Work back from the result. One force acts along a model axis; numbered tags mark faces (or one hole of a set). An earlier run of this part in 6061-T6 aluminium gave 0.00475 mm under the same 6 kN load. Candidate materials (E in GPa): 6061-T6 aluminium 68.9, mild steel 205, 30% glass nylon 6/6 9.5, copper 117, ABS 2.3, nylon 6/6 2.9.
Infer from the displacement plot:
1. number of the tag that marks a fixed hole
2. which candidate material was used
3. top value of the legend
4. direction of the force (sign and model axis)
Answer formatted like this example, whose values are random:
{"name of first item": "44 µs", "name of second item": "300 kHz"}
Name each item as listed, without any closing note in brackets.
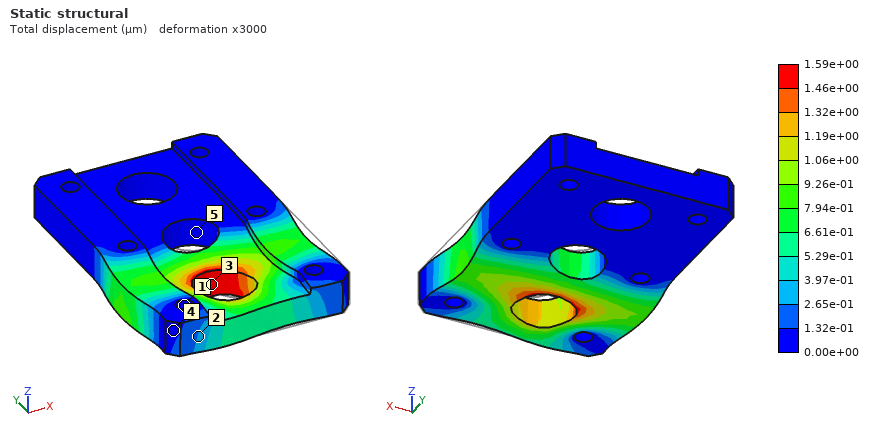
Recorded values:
{"number of the tag that marks a fixed hole": "1", "which candidate material was used": "mild steel", "top value of the legend": "1.59e+00 µm", "direction of the force": "-X"}
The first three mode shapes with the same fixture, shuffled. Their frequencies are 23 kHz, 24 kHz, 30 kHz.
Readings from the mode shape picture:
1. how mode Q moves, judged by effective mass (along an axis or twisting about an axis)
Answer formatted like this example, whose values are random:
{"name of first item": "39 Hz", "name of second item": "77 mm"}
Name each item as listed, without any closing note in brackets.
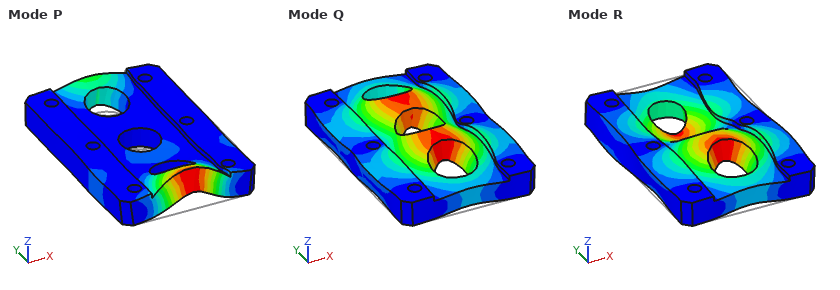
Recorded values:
{"how mode Q moves, judged by effective mass": "along Z"}
